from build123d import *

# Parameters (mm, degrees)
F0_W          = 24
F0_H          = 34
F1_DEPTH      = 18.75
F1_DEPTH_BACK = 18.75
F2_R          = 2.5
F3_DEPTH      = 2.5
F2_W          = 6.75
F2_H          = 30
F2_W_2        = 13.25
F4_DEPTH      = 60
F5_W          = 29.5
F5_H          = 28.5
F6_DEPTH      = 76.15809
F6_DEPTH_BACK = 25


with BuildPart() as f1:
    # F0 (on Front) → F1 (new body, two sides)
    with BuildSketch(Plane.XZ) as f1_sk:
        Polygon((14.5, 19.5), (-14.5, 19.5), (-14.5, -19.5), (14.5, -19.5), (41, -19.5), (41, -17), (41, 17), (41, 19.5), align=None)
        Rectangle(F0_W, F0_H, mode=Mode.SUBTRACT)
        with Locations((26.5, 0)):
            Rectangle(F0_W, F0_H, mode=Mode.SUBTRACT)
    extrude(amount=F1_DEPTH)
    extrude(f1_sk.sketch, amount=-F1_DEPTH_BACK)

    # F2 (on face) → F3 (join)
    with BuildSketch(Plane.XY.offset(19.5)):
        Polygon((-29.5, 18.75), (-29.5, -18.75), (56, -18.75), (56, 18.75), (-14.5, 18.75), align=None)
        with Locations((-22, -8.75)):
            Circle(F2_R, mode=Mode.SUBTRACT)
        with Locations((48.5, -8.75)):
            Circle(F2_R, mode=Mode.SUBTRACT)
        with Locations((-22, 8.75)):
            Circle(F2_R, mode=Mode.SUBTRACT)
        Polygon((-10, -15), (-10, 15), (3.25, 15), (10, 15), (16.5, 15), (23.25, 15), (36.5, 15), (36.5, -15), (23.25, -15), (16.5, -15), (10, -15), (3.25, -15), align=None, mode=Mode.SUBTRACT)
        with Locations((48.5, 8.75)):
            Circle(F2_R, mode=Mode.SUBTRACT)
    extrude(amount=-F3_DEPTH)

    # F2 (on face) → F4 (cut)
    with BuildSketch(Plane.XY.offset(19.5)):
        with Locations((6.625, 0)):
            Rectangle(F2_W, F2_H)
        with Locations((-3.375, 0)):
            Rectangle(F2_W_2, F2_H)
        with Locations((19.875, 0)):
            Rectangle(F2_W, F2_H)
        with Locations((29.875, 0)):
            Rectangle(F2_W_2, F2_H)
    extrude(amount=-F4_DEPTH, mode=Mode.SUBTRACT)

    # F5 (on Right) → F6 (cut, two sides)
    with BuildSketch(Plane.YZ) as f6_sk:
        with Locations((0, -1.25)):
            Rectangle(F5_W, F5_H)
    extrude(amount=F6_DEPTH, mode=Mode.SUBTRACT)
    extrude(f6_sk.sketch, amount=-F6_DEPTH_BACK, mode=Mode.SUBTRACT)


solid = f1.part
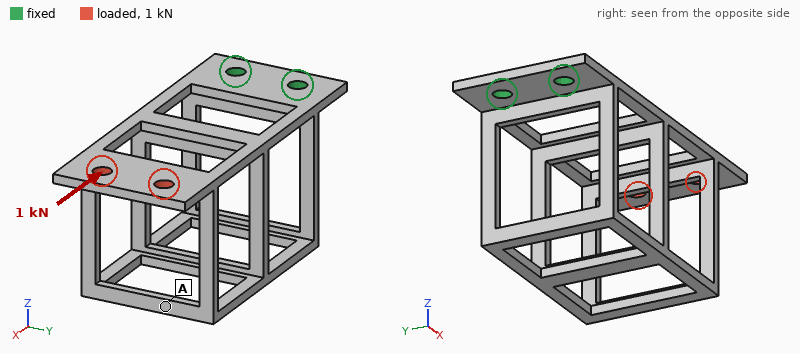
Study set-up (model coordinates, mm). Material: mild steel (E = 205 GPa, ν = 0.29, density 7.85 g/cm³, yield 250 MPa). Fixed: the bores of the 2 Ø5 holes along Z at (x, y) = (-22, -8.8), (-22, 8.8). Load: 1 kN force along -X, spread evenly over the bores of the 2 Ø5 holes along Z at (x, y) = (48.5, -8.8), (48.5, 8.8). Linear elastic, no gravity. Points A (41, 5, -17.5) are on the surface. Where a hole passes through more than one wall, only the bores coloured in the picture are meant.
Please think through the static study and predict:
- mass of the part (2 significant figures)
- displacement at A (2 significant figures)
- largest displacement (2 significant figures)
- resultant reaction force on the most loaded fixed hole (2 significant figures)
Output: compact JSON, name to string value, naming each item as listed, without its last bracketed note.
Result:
{"mass of the part": "81 g", "displacement at A": "10 µm", "largest displacement": "27 µm", "resultant reaction force on the most loaded fixed hole": "530 N"}
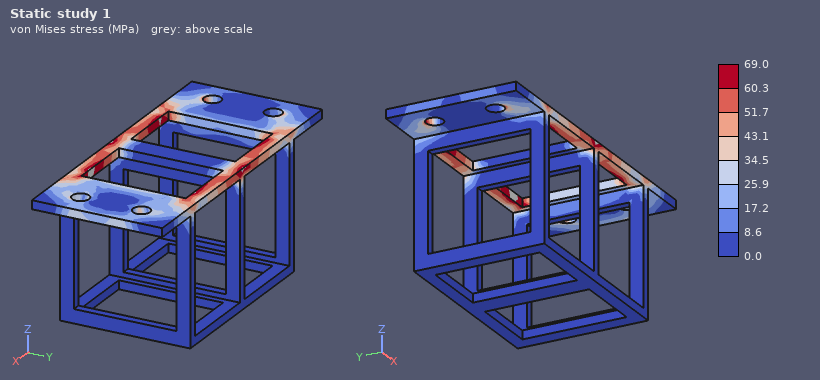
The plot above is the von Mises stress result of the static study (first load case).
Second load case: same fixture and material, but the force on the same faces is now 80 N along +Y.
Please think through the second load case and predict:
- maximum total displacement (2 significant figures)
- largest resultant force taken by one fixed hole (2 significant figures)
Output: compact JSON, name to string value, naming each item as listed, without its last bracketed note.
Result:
{"maximum total displacement": "64 µm", "largest resultant force taken by one fixed hole": "240 N"}
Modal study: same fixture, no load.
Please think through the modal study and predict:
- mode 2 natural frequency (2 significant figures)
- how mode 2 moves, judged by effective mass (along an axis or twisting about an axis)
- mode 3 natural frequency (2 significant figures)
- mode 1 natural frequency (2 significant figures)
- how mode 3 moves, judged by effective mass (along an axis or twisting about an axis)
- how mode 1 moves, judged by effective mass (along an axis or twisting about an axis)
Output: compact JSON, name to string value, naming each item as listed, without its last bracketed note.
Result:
{"mode 2 natural frequency": "800 Hz", "how mode 2 moves, judged by effective mass": "along Y", "mode 3 natural frequency": "1200 Hz", "mode 1 natural frequency": "250 Hz", "how mode 3 moves, judged by effective mass": "along Y", "how mode 1 moves, judged by effective mass": "along Z"}
